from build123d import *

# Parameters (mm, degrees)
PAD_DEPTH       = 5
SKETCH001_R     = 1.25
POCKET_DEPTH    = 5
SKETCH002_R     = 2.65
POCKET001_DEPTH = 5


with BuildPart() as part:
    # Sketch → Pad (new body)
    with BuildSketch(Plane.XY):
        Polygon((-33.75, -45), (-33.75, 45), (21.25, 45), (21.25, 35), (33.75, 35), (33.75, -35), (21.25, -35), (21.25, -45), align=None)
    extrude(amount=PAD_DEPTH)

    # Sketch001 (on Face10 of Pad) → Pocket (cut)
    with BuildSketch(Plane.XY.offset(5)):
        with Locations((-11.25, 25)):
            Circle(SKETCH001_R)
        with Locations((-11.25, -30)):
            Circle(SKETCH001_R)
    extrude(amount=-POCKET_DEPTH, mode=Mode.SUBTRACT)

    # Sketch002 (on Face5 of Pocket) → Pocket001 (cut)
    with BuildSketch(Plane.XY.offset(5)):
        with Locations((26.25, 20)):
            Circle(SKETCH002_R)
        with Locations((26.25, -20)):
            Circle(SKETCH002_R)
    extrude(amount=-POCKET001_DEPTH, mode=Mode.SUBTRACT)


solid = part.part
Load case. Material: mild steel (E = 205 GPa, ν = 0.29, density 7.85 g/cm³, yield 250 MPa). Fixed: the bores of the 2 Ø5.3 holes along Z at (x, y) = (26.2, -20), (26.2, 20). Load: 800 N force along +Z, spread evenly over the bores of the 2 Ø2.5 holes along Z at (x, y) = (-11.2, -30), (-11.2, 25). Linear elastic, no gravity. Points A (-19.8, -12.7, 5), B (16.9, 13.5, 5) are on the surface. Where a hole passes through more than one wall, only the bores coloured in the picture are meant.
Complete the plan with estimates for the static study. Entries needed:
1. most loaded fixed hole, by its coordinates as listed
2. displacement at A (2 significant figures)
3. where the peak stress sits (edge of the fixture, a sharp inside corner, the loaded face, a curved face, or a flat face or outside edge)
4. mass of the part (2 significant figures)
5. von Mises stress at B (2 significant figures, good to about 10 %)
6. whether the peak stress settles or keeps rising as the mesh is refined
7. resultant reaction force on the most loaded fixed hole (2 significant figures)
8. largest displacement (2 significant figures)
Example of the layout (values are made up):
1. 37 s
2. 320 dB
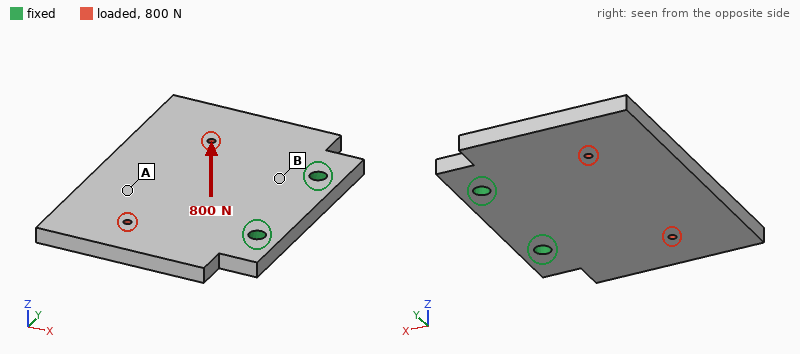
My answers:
1. (26.2, -20)
2. 0.13 mm
3. edge of the fixture
4. 230 g
5. 64 MPa
6. keeps rising
7. 440 N
8. 0.19 mm
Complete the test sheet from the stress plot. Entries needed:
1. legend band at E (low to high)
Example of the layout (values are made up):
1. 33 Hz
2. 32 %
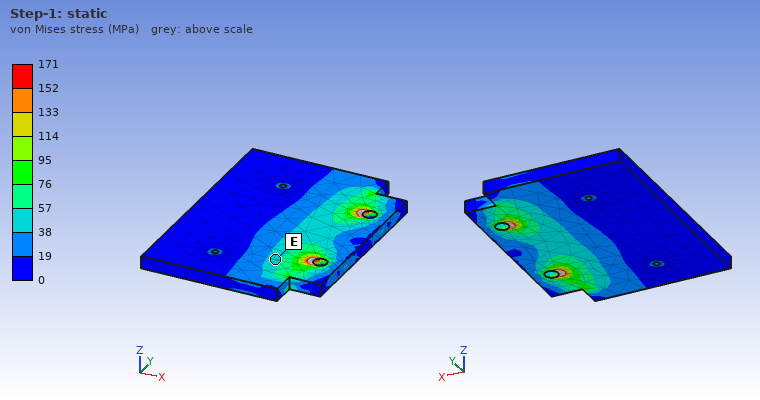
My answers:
1. 38 to 57 MPa
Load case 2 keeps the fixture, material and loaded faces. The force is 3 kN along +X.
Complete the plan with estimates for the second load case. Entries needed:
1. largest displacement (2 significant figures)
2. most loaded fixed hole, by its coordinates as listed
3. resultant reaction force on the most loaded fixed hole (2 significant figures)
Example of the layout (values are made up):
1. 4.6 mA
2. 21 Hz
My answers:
1. 3.4 µm
2. (26.2, -20)
3. 1.7 kN
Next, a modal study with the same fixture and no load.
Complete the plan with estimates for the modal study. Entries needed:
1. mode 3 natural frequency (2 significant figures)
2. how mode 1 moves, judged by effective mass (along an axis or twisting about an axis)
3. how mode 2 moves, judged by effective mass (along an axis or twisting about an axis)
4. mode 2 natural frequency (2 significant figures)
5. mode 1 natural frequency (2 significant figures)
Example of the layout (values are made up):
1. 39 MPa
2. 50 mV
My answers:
1. 4000 Hz
2. along Z
3. twisting about X
4. 1800 Hz
5. 1000 Hz
